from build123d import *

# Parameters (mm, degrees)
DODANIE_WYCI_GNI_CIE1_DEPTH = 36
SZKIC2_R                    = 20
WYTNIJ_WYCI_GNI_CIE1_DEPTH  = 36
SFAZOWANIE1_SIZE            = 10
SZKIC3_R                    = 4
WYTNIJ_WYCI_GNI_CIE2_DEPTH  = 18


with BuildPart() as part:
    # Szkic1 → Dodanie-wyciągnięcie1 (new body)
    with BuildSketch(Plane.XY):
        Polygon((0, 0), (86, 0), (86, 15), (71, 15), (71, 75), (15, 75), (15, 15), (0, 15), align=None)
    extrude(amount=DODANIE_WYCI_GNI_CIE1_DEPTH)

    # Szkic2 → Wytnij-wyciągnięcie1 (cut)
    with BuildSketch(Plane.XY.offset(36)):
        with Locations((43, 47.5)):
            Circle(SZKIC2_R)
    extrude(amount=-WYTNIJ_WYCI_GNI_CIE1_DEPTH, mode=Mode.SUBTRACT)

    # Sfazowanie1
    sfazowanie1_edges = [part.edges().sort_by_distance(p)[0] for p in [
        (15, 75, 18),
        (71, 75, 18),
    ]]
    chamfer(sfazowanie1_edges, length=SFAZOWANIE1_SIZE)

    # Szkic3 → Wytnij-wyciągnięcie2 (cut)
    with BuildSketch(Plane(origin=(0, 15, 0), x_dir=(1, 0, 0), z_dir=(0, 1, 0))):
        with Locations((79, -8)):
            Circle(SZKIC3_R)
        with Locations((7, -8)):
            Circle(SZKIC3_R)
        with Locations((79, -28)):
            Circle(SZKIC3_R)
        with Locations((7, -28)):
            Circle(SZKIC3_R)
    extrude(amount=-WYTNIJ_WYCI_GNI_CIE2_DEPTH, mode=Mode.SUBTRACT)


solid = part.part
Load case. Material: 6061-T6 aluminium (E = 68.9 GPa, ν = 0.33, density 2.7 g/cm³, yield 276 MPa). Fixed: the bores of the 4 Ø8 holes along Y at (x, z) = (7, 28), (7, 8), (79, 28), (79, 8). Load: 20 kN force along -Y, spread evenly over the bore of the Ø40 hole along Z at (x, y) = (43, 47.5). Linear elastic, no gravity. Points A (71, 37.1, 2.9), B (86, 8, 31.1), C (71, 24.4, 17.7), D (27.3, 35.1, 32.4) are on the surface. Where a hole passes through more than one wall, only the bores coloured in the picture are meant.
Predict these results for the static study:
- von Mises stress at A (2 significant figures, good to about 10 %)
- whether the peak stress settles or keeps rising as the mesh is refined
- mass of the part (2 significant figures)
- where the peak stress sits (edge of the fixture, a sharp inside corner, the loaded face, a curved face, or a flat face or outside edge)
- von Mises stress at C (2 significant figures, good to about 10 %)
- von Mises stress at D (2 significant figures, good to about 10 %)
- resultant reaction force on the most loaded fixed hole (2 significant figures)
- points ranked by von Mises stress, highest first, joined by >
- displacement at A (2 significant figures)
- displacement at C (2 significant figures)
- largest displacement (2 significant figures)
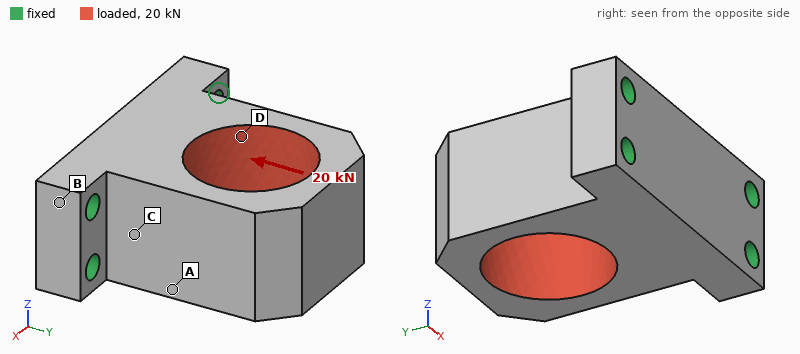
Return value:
24 MPa
keeps rising
310 g
edge of the fixture
32 MPa
13 MPa
5.3 kN
C > A > D > B
20 µm
14 µm
43 µm
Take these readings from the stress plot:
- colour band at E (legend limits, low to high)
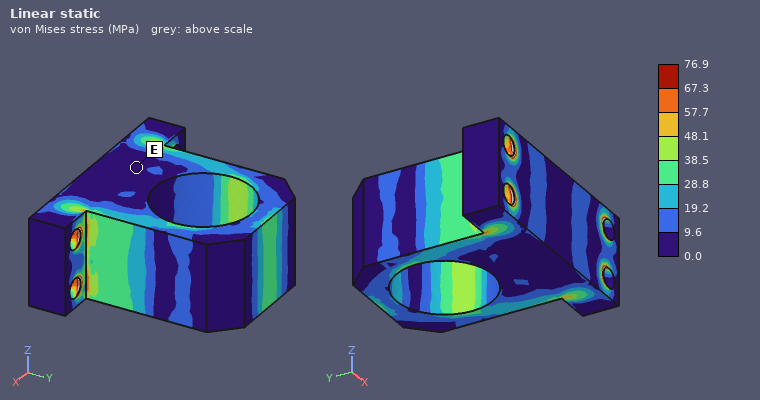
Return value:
0.0 to 9.6 MPa
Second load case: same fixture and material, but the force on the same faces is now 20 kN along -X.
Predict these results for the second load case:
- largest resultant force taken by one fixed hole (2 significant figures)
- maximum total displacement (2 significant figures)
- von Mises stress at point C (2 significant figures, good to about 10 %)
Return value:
8.3 kN
0.19 mm
73 MPa
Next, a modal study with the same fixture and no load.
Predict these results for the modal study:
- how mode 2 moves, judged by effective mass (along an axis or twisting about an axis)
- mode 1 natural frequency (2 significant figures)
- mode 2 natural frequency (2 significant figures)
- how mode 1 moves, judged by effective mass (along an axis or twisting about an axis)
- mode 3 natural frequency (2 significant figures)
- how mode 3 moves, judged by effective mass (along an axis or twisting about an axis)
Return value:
along X
3500 Hz
4600 Hz
along Z
7500 Hz
twisting about Y
